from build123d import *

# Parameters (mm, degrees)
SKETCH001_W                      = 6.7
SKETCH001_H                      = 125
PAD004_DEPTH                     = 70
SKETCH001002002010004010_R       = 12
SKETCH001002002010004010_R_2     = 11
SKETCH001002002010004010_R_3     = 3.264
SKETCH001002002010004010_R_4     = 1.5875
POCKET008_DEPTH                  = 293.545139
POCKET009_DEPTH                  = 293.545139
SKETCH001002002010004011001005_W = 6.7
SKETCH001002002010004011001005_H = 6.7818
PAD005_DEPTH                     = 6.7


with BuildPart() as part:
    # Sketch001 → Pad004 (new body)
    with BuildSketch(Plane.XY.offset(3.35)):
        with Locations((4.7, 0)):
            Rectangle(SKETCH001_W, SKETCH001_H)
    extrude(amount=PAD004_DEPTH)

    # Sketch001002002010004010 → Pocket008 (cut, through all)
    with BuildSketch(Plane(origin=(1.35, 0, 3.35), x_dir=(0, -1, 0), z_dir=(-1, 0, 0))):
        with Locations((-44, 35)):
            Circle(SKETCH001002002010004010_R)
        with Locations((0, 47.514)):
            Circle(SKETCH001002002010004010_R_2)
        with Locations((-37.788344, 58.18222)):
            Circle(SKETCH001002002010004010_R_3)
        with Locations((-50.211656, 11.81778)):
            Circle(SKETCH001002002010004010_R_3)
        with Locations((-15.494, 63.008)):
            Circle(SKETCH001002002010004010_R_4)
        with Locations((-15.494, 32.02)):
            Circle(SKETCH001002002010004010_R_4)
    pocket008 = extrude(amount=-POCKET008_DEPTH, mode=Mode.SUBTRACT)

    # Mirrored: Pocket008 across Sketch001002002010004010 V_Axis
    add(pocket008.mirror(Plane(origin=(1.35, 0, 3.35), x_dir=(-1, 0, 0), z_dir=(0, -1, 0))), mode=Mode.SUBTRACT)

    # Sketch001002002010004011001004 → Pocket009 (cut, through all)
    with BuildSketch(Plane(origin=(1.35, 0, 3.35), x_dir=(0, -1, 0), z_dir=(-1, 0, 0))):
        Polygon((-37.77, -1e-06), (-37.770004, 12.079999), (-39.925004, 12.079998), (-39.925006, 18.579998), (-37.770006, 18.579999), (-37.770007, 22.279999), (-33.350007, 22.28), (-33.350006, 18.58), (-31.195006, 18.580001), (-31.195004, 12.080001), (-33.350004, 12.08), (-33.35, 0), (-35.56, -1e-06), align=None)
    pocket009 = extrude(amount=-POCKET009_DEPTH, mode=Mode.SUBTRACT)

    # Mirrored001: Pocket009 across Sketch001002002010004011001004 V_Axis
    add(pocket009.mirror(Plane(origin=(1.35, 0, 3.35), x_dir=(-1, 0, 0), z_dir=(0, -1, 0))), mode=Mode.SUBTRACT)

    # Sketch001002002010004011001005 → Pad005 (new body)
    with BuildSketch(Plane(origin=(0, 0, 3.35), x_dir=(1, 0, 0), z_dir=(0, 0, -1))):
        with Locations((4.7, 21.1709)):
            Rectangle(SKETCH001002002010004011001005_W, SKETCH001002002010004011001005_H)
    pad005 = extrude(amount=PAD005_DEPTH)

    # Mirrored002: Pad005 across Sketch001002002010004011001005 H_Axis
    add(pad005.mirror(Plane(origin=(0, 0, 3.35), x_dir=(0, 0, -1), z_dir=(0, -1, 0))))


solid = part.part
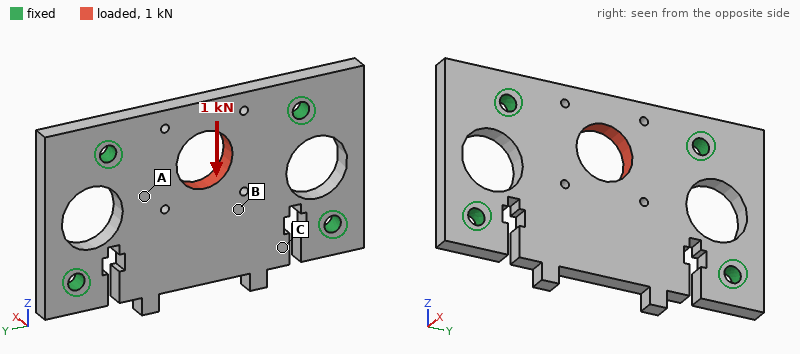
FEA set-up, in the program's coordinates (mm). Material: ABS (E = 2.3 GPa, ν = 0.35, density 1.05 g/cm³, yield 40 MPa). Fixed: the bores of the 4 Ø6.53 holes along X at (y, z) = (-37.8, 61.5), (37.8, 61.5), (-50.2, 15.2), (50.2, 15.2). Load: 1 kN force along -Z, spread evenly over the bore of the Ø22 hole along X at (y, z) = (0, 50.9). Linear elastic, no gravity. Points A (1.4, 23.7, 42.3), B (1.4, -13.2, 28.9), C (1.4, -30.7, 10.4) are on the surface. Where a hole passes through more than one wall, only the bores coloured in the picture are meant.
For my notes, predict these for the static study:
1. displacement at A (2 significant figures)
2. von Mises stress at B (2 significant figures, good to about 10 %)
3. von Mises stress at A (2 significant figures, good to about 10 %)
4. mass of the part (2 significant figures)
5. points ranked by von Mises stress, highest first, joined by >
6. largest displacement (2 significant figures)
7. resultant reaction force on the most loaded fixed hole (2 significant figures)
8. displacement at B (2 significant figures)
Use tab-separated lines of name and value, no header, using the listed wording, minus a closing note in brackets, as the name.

displacement at A	0.061 mm
von Mises stress at B	2.1 MPa
von Mises stress at A	3.6 MPa
mass of the part	50 g
points ranked by von Mises stress, highest first, joined by >	A > B > C
largest displacement	0.13 mm
resultant reaction force on the most loaded fixed hole	480 N
displacement at B	0.070 mm
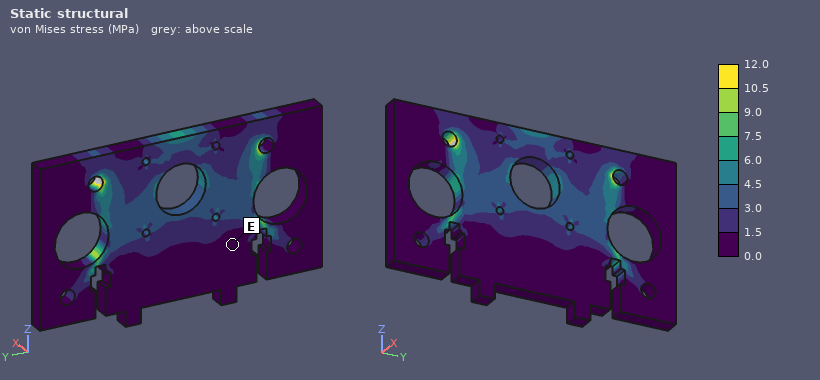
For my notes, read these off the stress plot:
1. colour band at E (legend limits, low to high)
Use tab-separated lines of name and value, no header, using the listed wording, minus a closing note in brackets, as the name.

colour band at E	0.0 to 1.5 MPa
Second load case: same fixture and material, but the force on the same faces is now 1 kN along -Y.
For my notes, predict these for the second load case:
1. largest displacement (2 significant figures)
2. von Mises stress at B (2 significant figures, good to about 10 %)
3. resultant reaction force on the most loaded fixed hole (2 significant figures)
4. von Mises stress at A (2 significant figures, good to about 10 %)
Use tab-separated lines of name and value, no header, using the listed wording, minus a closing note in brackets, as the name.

largest displacement	51 µm
von Mises stress at B	0.56 MPa
resultant reaction force on the most loaded fixed hole	430 N
von Mises stress at A	1.2 MPa
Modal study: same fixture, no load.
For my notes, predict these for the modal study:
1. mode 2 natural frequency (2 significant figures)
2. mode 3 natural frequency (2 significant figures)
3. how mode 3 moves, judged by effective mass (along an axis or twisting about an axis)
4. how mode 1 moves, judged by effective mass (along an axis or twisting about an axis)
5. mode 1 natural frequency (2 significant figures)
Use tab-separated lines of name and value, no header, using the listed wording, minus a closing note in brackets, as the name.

mode 2 natural frequency	1500 Hz
mode 3 natural frequency	1700 Hz
how mode 3 moves, judged by effective mass	along X
how mode 1 moves, judged by effective mass	along X
mode 1 natural frequency	580 Hz
